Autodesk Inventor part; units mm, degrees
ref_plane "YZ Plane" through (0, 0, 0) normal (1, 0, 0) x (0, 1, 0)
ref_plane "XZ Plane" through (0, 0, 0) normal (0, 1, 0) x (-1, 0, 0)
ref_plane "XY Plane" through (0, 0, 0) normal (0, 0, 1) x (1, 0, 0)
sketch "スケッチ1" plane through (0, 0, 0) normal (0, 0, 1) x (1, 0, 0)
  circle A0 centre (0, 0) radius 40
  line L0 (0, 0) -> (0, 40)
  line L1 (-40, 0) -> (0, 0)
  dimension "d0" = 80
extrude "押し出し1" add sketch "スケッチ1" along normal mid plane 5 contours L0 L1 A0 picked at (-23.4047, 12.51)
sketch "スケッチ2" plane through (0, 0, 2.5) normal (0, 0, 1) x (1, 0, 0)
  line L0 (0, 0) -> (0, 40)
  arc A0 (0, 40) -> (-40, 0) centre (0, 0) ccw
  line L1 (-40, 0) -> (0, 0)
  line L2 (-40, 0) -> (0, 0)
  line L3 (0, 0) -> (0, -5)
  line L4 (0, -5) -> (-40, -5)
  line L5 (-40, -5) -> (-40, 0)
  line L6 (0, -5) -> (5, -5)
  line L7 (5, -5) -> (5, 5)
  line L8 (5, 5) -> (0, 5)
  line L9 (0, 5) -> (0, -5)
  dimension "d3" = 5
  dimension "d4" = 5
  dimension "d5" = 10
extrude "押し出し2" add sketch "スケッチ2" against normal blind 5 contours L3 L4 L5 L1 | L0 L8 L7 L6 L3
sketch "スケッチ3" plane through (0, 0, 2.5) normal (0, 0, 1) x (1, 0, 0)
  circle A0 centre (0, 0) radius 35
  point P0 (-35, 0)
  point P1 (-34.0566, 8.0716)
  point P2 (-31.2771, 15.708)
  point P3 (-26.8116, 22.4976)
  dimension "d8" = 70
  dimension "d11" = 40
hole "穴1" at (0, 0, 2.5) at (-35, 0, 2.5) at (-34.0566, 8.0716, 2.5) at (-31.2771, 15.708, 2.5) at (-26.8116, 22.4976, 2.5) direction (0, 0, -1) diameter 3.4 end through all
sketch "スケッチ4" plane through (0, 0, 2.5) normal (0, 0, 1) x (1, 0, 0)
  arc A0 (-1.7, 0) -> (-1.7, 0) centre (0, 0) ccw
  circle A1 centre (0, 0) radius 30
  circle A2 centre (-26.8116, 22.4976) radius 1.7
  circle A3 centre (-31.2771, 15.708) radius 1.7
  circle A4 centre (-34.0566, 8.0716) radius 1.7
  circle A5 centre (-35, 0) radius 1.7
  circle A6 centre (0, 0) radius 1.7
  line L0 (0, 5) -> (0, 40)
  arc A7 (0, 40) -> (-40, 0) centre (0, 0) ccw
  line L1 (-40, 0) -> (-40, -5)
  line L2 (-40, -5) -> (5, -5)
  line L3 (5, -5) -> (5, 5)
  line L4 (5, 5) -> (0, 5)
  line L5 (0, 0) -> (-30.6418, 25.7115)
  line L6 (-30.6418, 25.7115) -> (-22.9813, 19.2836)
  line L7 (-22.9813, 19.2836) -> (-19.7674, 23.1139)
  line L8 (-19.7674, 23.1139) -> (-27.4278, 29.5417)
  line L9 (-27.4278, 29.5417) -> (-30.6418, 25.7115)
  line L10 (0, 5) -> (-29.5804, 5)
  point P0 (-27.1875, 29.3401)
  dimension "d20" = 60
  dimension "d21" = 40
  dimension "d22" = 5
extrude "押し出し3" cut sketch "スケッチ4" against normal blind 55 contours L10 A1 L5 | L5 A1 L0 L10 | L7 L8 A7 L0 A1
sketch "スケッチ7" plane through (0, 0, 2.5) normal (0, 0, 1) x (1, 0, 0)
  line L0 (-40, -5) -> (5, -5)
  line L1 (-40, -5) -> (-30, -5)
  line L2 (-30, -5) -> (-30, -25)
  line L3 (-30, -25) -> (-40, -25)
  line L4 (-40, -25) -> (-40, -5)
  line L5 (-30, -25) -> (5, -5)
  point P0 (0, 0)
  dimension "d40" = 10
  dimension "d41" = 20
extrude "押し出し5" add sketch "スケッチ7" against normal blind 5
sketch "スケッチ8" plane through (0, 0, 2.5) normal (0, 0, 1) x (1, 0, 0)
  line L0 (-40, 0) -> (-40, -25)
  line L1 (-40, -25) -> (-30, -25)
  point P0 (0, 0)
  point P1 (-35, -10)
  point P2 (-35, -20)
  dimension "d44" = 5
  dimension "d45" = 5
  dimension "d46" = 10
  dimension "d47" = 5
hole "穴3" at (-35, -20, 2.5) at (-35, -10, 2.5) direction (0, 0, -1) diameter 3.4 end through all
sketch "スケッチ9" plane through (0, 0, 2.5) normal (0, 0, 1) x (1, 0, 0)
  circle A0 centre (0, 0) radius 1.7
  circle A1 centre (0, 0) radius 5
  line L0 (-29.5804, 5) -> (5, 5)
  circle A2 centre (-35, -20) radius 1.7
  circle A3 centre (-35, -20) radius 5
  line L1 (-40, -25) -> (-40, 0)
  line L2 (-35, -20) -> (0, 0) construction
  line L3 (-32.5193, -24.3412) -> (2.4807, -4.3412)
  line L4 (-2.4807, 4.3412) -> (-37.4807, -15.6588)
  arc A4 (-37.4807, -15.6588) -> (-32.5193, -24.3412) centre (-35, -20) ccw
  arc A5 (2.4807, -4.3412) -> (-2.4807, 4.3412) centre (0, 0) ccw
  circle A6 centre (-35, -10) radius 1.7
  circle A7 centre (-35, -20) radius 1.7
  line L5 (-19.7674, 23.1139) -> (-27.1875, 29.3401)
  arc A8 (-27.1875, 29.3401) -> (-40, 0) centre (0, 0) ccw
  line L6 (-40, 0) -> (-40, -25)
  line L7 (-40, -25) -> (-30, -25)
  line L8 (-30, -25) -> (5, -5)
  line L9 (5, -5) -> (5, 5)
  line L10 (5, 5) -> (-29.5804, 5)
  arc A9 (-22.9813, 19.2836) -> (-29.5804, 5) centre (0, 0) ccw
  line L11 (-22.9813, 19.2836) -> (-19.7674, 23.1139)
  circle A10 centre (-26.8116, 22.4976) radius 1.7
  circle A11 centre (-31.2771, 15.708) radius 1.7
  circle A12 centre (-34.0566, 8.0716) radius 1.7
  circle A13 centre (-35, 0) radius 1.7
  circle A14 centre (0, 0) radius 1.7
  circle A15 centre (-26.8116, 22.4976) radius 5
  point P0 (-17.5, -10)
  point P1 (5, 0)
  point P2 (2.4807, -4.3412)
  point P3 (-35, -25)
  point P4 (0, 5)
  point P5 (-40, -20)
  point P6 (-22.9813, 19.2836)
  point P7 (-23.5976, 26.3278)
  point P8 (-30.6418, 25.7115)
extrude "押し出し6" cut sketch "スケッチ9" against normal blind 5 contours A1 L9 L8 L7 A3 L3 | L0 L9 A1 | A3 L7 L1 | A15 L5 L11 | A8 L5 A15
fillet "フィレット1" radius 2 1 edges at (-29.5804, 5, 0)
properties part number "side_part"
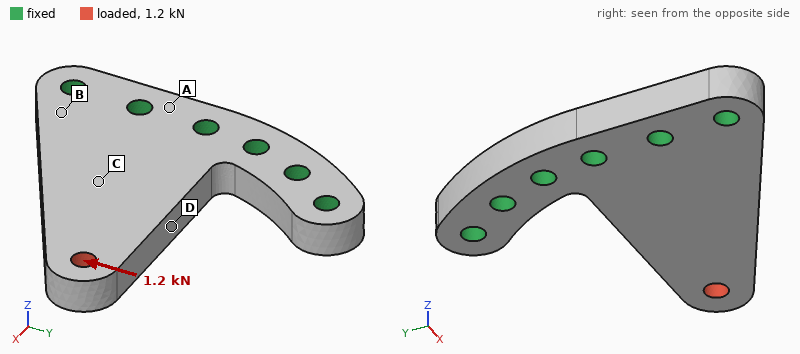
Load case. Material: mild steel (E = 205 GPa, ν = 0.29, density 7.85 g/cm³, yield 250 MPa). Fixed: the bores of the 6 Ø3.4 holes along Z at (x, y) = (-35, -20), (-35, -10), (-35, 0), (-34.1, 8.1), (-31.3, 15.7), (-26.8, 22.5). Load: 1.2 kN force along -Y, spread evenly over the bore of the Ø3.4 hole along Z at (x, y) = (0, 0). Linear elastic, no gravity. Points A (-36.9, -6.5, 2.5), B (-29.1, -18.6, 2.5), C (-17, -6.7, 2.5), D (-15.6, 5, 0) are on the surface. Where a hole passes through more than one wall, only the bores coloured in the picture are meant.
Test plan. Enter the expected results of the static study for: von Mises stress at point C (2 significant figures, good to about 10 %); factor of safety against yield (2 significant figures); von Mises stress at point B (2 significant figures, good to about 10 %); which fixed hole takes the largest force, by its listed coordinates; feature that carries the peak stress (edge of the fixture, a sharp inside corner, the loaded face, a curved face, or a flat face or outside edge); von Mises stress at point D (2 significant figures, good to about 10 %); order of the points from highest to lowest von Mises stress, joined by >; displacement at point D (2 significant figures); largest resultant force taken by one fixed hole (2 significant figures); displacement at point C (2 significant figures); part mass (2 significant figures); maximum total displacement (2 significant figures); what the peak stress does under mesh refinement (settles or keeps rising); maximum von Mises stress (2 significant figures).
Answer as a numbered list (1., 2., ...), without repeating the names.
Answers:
1. 23 MPa
2. 1.8
3. 44 MPa
4. (-35, -20)
5. a curved face
6. 63 MPa
7. D > B > C > A
8. 8.3 µm
9. 1.6 kN
10. 4.7 µm
11. 42 g
12. 26 µm
13. settles
14. 140 MPa
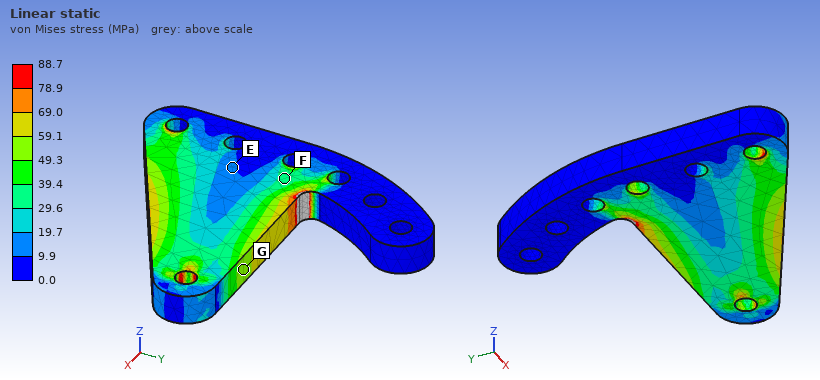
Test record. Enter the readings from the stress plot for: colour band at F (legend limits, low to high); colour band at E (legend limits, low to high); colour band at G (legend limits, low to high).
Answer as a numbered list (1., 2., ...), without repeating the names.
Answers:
1. 29.6 to 39.4 MPa
2. 9.9 to 19.7 MPa
3. 49.3 to 59.1 MPa
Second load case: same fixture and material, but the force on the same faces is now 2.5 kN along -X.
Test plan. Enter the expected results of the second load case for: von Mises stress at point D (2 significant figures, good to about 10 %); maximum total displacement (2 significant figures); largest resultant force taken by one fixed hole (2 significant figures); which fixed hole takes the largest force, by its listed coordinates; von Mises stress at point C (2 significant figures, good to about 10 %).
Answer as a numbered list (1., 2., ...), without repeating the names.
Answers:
1. 63 MPa
2. 14 µm
3. 1.4 kN
4. (-35, 0)
5. 18 MPa
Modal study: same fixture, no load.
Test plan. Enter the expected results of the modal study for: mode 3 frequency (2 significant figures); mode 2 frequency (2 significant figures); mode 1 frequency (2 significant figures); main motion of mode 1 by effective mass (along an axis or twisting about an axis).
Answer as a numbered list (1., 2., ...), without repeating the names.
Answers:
1. 16 kHz
2. 16 kHz
3. 3900 Hz
4. along Z
